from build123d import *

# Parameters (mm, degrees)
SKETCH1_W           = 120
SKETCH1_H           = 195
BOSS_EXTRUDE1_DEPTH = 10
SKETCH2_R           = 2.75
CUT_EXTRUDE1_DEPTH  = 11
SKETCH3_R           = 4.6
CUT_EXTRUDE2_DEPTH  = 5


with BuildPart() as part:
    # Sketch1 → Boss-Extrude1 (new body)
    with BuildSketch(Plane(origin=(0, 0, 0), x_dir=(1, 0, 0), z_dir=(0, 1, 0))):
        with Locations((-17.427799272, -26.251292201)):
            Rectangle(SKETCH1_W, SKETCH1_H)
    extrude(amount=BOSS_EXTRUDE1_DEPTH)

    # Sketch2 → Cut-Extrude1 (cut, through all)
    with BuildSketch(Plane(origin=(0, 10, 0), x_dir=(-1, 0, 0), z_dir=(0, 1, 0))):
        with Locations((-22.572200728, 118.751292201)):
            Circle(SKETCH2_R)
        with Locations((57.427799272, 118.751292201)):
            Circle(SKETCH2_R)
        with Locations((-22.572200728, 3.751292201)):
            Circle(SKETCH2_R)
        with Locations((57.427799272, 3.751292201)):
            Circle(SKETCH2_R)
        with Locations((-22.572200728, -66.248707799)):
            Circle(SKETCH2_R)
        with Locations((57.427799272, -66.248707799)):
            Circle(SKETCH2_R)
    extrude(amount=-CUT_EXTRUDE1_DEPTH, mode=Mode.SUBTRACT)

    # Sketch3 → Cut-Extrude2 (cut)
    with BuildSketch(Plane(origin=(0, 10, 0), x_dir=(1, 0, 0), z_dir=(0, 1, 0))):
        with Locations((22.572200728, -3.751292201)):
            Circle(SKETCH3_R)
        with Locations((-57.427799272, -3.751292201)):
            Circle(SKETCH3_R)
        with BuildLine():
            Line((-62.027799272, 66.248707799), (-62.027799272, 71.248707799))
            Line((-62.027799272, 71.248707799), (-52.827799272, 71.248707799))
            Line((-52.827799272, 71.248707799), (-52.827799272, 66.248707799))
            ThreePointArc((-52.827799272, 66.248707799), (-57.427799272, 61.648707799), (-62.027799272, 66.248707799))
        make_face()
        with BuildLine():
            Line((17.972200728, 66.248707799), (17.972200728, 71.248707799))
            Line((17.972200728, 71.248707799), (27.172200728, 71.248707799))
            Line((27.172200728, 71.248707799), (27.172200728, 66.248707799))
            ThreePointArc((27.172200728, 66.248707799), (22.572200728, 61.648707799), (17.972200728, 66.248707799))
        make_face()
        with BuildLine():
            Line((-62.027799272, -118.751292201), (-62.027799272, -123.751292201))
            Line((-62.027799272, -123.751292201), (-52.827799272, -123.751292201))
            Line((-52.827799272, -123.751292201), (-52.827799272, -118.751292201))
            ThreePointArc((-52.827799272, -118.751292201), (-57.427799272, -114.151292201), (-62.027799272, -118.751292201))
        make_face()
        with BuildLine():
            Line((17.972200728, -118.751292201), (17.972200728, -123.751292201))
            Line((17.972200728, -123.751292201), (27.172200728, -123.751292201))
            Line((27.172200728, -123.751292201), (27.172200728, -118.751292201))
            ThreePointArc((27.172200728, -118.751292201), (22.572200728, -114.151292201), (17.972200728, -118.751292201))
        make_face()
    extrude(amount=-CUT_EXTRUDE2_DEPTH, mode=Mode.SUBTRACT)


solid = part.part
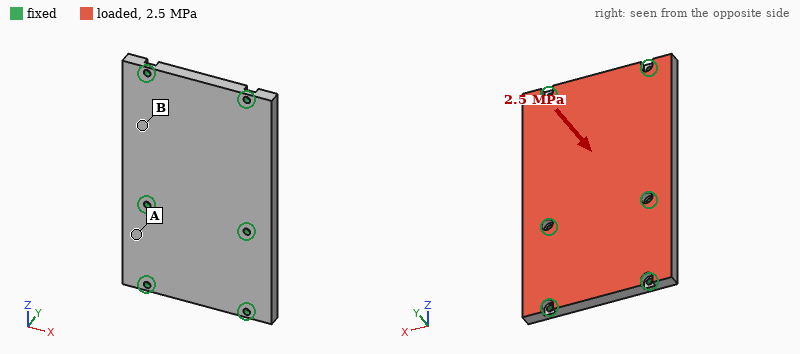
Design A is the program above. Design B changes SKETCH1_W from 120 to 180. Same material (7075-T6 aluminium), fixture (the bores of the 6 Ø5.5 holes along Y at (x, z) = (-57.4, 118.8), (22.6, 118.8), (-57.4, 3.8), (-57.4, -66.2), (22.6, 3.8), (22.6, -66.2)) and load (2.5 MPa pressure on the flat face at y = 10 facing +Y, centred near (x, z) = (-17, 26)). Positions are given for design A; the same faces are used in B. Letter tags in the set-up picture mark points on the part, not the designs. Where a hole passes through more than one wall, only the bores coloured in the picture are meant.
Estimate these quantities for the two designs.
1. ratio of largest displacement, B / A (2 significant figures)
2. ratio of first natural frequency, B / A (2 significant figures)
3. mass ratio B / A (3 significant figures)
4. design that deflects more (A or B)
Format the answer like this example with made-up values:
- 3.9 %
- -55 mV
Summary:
- 2.6
- 0.70
- 1.51
- B
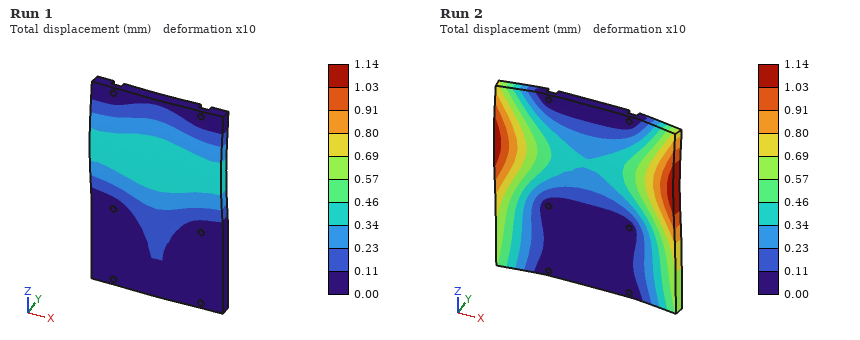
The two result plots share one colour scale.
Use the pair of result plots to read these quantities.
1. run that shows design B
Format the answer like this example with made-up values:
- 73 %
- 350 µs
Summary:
- Run 2
